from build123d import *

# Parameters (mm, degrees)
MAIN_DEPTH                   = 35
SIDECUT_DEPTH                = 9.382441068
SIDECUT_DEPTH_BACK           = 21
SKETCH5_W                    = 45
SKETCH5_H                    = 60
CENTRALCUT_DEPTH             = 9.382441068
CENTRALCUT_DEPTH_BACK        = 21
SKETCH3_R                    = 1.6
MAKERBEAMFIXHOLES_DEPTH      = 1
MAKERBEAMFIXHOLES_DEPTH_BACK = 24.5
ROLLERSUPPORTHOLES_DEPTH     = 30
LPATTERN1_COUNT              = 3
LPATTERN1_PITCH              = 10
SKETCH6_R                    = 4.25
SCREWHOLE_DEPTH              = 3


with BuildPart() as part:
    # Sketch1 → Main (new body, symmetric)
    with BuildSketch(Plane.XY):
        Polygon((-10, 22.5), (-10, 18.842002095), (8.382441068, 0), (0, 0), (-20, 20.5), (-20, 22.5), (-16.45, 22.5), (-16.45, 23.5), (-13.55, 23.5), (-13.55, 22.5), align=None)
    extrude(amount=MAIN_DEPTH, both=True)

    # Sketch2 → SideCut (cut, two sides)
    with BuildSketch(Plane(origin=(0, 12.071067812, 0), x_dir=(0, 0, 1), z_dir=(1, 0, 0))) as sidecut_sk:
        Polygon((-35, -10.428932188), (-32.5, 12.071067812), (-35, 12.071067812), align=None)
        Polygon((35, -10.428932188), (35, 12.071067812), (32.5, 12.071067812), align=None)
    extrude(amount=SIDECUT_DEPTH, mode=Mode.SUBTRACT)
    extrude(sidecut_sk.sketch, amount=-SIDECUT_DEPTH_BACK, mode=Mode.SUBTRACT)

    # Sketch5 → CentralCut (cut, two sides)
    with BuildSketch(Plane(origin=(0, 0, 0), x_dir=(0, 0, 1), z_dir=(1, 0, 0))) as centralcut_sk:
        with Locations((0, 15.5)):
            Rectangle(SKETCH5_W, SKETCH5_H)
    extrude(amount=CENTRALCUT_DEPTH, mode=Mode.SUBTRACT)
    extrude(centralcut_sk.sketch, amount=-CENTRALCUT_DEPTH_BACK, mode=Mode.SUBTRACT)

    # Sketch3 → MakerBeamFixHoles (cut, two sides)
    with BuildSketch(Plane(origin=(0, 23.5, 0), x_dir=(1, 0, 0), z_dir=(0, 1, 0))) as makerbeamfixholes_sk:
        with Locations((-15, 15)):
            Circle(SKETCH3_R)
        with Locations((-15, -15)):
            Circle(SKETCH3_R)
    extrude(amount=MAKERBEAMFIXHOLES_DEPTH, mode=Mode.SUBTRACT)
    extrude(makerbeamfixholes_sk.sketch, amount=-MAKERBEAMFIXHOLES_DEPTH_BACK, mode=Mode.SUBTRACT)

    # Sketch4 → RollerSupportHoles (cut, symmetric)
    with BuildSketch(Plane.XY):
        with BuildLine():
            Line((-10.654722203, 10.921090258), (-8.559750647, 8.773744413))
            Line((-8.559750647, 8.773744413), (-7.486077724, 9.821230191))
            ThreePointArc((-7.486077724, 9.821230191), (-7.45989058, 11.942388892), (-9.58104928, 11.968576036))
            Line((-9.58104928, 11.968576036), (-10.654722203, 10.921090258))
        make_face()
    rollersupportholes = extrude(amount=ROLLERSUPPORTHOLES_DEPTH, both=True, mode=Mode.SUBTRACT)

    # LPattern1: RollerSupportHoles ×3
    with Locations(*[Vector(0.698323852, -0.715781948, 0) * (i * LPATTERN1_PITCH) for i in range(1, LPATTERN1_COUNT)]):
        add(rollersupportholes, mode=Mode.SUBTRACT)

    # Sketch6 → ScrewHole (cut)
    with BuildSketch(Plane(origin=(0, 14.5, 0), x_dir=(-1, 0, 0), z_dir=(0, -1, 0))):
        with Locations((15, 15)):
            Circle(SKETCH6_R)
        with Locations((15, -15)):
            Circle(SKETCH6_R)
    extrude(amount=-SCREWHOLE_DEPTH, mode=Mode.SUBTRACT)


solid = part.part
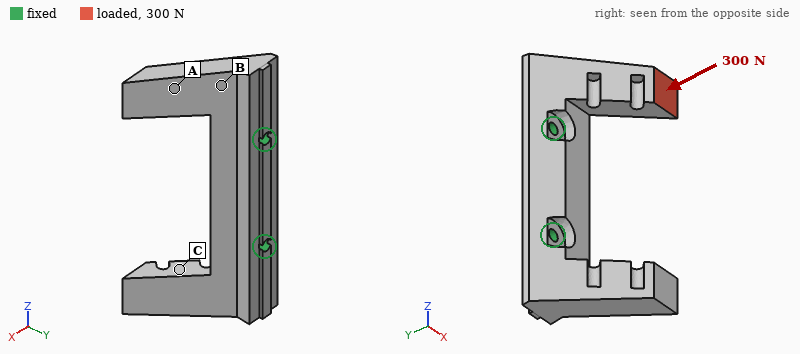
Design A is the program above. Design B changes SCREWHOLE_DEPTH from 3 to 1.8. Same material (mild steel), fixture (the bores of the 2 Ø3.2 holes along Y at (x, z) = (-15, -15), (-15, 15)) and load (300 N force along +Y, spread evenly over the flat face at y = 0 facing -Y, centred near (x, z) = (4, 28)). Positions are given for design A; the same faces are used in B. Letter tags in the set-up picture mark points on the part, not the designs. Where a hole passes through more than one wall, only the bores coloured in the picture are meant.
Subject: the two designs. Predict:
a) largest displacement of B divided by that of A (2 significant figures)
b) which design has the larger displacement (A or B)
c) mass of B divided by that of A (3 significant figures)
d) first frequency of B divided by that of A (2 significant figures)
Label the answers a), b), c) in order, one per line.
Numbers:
a) 0.88
b) A
c) 1.01
d) 1.1
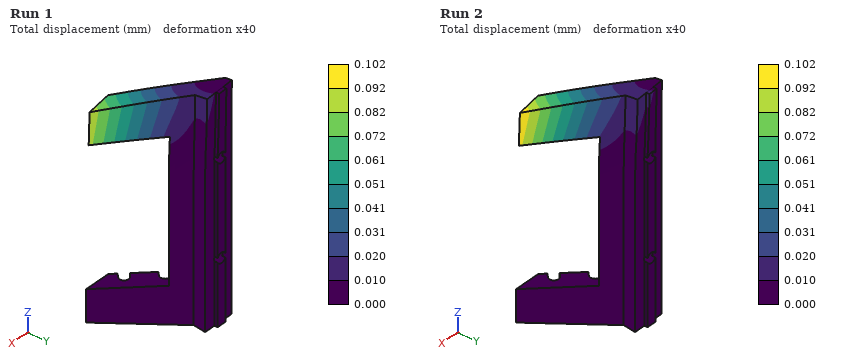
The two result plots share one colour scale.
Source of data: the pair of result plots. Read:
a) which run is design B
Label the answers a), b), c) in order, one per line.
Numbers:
a) Run 1
